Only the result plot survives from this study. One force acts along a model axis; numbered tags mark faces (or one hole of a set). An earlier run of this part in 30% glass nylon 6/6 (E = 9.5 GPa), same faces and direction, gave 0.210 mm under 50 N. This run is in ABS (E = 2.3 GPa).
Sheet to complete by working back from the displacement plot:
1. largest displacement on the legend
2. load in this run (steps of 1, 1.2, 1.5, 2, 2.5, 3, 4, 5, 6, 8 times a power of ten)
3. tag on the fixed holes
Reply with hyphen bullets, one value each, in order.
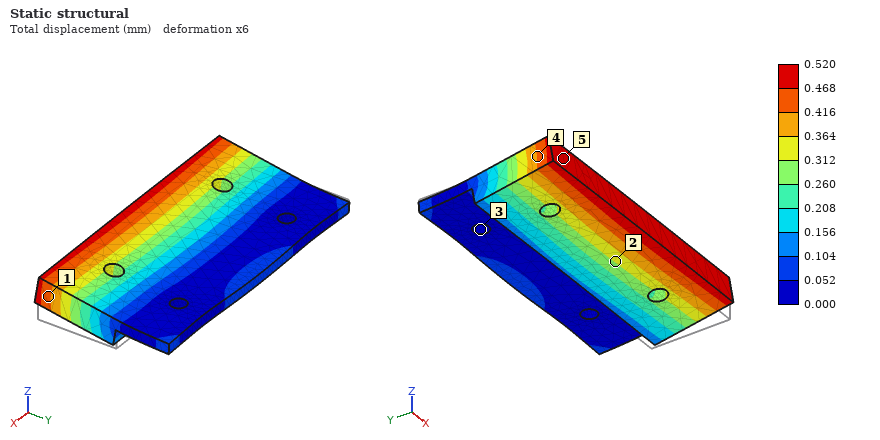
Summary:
- 0.520 mm
- 30 N
- 3
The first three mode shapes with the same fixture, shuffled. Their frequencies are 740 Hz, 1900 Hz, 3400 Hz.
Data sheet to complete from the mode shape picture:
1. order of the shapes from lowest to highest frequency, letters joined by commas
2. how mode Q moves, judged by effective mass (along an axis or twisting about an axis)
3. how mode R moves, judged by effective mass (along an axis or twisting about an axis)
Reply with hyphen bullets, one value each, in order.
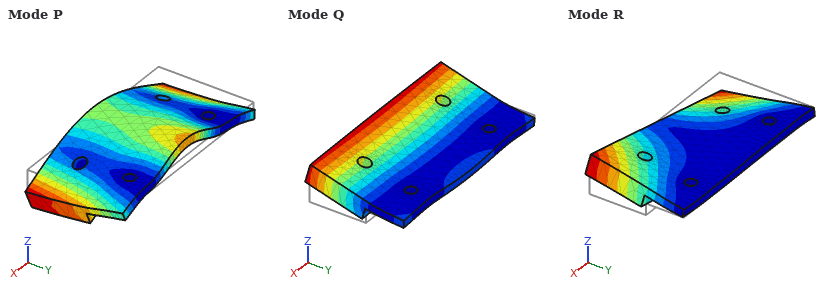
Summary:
- Q, R, P
- along Z
- twisting about Y
